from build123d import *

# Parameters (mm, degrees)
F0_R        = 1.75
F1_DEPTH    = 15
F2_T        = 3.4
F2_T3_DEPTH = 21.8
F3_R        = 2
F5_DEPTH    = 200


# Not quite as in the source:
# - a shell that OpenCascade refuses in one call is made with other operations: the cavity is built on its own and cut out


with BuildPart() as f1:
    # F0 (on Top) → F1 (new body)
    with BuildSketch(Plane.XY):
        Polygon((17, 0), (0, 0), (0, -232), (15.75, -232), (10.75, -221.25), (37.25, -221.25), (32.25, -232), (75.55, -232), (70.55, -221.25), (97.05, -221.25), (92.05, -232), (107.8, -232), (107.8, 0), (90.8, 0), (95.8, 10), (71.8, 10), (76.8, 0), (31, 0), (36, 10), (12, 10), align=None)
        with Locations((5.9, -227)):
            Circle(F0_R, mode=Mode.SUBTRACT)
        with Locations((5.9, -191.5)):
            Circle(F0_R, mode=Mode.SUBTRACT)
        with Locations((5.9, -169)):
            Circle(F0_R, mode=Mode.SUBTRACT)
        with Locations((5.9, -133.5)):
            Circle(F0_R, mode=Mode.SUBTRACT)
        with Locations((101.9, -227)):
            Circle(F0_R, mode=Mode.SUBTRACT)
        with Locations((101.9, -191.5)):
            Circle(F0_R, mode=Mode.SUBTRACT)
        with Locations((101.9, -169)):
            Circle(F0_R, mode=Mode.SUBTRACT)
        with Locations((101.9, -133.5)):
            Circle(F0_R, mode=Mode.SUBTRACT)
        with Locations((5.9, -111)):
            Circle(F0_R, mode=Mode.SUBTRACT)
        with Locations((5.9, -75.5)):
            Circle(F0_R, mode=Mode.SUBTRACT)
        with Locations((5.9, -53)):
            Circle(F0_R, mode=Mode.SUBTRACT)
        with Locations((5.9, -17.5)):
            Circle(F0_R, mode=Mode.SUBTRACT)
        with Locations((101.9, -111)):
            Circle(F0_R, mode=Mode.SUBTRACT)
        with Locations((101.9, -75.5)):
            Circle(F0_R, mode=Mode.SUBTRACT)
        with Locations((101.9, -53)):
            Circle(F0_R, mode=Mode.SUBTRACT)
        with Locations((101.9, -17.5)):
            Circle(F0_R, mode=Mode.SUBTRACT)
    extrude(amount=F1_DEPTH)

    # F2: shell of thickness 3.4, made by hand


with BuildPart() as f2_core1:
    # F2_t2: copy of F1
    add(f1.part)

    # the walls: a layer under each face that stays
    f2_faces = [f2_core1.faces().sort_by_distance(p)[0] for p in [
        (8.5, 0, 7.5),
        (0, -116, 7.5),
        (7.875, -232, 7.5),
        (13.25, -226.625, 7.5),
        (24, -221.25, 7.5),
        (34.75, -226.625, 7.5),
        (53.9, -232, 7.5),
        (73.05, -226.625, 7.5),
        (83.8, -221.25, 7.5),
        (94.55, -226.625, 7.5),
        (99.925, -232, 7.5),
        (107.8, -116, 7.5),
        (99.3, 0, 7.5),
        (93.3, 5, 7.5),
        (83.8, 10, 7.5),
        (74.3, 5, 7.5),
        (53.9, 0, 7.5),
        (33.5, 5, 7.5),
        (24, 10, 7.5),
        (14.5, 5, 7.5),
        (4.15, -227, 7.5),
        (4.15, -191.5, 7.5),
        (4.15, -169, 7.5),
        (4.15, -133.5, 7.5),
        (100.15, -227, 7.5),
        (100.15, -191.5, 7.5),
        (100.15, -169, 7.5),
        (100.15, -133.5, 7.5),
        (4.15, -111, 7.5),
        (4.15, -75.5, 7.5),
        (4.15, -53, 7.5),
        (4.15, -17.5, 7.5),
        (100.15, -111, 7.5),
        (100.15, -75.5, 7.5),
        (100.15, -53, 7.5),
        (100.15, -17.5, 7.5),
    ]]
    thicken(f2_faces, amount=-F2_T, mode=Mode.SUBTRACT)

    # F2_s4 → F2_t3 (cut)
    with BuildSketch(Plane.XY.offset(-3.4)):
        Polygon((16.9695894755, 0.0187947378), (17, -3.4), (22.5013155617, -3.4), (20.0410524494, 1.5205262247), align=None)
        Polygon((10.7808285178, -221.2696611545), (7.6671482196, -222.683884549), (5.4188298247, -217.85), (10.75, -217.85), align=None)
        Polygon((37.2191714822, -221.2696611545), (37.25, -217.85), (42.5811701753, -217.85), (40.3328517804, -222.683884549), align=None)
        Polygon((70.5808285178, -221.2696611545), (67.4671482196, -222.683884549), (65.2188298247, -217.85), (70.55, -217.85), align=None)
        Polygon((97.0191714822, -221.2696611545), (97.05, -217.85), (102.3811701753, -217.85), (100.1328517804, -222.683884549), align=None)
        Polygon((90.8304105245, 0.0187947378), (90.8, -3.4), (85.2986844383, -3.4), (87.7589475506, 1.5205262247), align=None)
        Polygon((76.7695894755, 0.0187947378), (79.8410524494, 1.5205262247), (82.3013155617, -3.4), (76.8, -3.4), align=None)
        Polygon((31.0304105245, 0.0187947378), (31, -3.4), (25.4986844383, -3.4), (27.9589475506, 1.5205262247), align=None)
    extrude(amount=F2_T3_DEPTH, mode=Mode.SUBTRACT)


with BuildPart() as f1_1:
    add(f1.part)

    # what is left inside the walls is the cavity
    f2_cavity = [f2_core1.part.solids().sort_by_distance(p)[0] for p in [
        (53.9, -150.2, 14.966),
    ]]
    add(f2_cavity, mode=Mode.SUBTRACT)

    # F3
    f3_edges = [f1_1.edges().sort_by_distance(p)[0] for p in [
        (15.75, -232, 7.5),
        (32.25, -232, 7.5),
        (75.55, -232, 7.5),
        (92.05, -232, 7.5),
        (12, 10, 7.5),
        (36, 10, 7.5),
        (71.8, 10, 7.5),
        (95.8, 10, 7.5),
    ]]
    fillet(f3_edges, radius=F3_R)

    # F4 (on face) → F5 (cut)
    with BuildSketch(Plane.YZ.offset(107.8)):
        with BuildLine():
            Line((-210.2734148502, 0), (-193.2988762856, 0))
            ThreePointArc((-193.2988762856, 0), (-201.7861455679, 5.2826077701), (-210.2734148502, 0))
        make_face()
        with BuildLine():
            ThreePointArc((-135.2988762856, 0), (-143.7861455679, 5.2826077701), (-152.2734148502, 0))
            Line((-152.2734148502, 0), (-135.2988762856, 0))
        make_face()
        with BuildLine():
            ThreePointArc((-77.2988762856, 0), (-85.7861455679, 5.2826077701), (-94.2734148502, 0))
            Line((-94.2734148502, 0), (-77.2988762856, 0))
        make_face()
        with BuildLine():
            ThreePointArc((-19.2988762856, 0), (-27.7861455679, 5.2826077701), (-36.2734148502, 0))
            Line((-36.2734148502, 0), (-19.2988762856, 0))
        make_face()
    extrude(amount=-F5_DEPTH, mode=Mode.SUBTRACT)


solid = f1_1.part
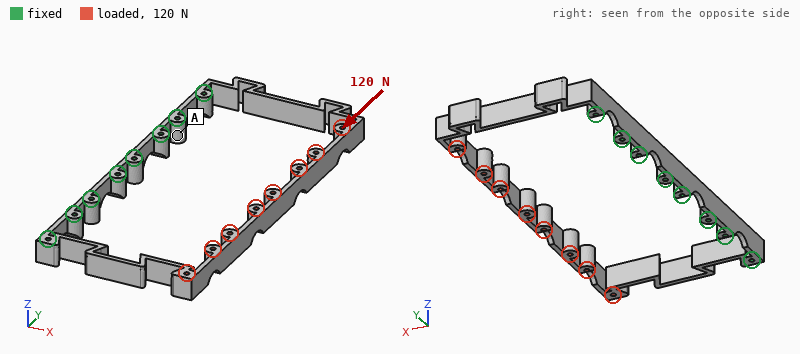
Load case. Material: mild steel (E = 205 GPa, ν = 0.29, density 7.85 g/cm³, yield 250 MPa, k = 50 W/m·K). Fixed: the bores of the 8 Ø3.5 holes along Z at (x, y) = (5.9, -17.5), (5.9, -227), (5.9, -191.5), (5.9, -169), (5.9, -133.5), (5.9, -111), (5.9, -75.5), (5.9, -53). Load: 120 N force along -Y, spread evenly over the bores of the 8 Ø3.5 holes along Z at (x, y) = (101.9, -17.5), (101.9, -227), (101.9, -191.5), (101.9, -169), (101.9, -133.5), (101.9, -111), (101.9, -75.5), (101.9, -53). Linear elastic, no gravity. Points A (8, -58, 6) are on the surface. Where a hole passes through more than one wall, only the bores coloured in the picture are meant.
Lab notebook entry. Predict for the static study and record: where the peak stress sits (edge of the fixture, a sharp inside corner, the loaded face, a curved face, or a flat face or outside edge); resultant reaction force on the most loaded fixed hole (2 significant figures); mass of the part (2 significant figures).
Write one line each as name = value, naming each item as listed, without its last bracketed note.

where the peak stress sits = a curved face
resultant reaction force on the most loaded fixed hole = 120 N
mass of the part = 400 g
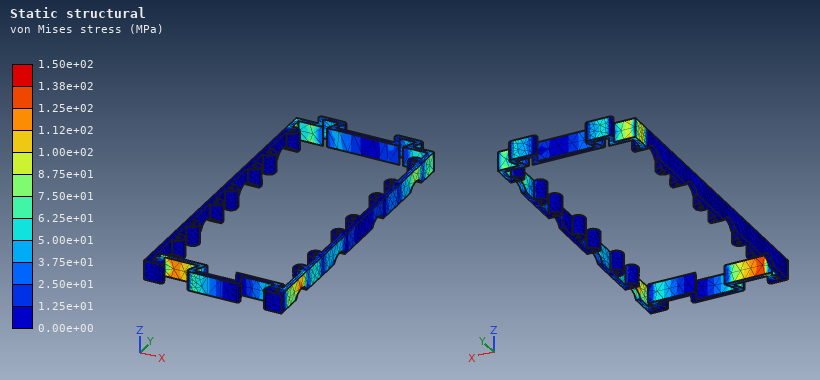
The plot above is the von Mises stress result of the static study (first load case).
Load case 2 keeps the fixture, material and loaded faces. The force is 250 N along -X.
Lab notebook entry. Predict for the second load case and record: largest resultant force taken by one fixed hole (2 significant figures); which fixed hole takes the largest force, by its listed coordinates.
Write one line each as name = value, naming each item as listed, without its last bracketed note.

largest resultant force taken by one fixed hole = 170 N
which fixed hole takes the largest force, by its listed coordinates = (5.9, -17.5)
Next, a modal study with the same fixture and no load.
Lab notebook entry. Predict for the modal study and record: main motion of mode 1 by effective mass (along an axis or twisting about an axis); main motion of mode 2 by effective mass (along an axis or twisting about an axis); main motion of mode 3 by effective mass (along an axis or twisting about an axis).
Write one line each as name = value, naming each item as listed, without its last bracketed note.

main motion of mode 1 by effective mass = along Y
main motion of mode 2 by effective mass = along Z
main motion of mode 3 by effective mass = along X
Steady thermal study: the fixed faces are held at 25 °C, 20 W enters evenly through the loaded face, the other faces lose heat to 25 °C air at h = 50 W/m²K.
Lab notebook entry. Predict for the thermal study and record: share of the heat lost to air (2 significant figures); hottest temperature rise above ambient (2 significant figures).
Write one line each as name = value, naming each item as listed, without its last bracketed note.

share of the heat lost to air = 99 %
hottest temperature rise above ambient = 40 K
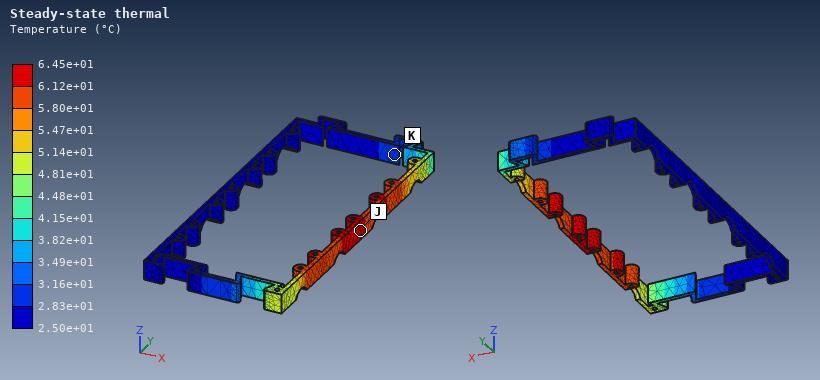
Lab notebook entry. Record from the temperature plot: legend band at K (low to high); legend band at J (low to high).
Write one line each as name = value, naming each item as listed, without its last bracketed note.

legend band at K = 2.83e+01 to 3.16e+01 °C
legend band at J = 6.12e+01 to 6.45e+01 °C
